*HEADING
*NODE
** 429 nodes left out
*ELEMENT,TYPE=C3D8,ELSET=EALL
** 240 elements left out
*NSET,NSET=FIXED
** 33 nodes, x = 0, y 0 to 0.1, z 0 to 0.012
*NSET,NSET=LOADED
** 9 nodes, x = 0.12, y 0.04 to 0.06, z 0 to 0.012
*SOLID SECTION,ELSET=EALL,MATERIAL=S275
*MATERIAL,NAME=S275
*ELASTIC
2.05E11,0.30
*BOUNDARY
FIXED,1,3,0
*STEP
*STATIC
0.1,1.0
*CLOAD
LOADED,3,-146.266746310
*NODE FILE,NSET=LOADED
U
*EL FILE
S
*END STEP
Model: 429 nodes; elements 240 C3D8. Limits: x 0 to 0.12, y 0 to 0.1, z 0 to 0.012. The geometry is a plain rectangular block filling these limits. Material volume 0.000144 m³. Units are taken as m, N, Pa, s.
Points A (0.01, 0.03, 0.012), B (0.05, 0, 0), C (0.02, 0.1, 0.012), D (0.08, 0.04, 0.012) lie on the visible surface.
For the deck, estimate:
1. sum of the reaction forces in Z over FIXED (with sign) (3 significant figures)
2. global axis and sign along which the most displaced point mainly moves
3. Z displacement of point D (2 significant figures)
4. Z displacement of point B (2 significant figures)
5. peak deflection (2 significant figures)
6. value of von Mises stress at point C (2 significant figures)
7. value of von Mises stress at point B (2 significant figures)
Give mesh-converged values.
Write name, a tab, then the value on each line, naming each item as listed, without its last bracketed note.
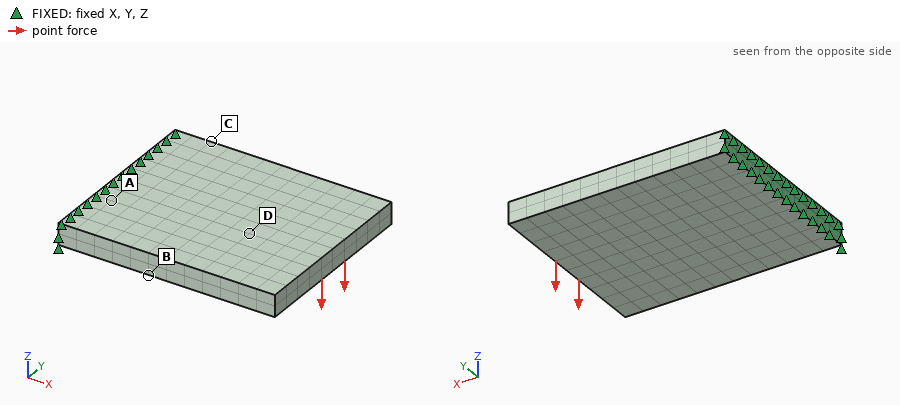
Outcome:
sum of the reaction forces in Z over FIXED (with sign)	1320 N
global axis and sign along which the most displaced point mainly moves	-Z
Z displacement of point D	-1.3e-04 m
Z displacement of point B	-4.9e-05 m
peak deflection	2.5e-04 m
value of von Mises stress at point C	5.3e+07 Pa
value of von Mises stress at point B	3.9e+07 Pa
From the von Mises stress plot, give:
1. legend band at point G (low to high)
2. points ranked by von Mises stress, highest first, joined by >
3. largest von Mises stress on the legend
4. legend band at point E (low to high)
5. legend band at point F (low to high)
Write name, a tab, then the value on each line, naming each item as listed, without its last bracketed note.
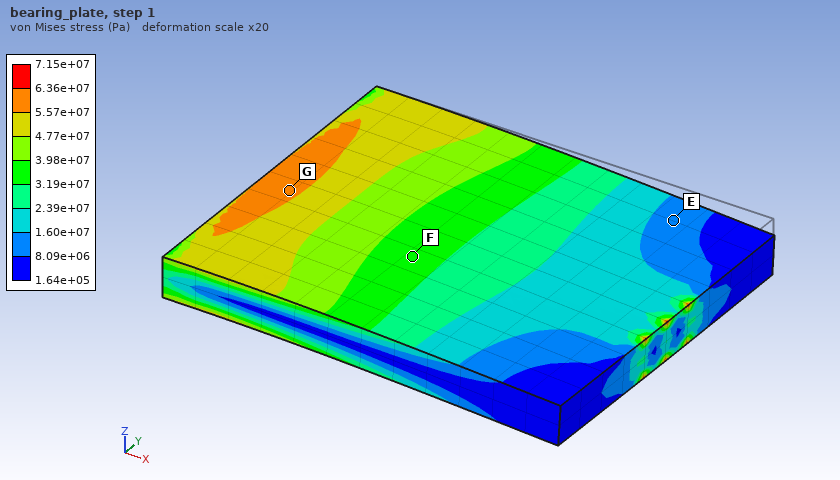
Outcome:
legend band at point G	5.57e+07 to 6.36e+07 Pa
points ranked by von Mises stress, highest first, joined by >	G > F > E
largest von Mises stress on the legend	7.15e+07 Pa
legend band at point E	8.09e+06 to 1.60e+07 Pa
legend band at point F	3.19e+07 to 3.98e+07 Pa
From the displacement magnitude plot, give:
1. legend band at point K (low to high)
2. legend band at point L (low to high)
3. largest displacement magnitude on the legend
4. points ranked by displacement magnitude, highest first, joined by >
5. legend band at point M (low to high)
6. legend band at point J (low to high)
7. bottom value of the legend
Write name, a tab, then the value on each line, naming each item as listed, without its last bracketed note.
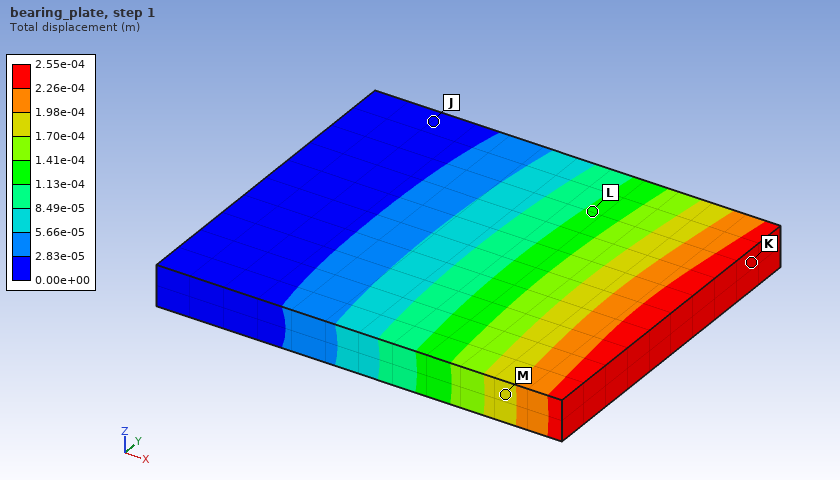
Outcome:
legend band at point K	2.26e-04 to 2.55e-04 m
legend band at point L	1.13e-04 to 1.41e-04 m
largest displacement magnitude on the legend	2.55e-04 m
points ranked by displacement magnitude, highest first, joined by >	K > M > L > J
legend band at point M	1.70e-04 to 1.98e-04 m
legend band at point J	0.00e+00 to 2.83e-05 m
bottom value of the legend	0.00e+00 m
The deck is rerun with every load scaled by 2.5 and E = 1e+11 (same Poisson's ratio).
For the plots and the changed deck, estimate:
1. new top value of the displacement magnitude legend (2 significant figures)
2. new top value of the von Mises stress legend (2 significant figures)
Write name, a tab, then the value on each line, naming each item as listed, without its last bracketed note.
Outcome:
new top value of the displacement magnitude legend	0.0013 m
new top value of the von Mises stress legend	1.8e+08 Pa
